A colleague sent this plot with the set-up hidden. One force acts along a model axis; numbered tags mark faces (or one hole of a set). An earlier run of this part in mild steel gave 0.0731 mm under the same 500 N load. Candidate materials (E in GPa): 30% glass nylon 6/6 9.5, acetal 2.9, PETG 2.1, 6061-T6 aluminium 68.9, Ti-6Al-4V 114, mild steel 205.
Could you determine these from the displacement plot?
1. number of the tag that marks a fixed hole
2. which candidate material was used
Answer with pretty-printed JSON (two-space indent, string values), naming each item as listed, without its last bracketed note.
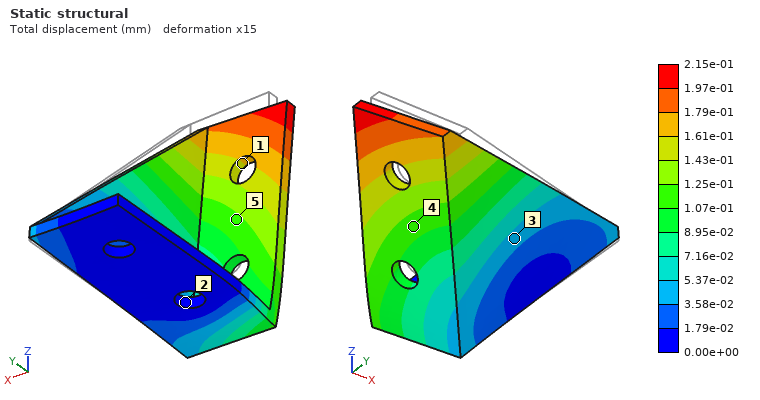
{
  "number of the tag that marks a fixed hole": "2",
  "which candidate material was used": "6061-T6 aluminium"
}
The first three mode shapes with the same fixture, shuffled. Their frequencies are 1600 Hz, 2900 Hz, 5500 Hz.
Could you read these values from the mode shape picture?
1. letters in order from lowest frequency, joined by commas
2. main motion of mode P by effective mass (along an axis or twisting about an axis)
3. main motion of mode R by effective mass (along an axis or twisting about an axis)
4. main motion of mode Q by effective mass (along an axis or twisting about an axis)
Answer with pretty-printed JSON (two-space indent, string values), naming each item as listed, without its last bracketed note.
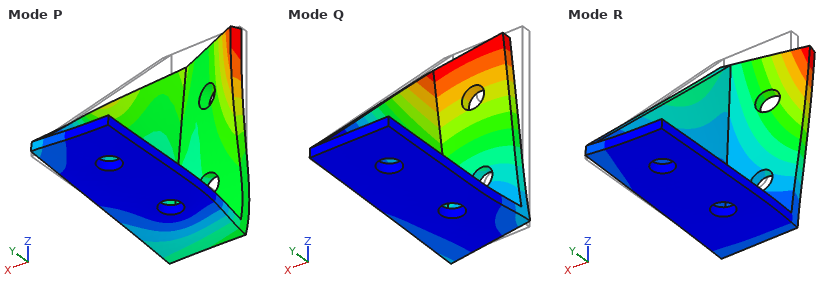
{
  "letters in order from lowest frequency, joined by commas": "Q, R, P",
  "main motion of mode P by effective mass": "along Z",
  "main motion of mode R by effective mass": "along Y",
  "main motion of mode Q by effective mass": "along X"
}
